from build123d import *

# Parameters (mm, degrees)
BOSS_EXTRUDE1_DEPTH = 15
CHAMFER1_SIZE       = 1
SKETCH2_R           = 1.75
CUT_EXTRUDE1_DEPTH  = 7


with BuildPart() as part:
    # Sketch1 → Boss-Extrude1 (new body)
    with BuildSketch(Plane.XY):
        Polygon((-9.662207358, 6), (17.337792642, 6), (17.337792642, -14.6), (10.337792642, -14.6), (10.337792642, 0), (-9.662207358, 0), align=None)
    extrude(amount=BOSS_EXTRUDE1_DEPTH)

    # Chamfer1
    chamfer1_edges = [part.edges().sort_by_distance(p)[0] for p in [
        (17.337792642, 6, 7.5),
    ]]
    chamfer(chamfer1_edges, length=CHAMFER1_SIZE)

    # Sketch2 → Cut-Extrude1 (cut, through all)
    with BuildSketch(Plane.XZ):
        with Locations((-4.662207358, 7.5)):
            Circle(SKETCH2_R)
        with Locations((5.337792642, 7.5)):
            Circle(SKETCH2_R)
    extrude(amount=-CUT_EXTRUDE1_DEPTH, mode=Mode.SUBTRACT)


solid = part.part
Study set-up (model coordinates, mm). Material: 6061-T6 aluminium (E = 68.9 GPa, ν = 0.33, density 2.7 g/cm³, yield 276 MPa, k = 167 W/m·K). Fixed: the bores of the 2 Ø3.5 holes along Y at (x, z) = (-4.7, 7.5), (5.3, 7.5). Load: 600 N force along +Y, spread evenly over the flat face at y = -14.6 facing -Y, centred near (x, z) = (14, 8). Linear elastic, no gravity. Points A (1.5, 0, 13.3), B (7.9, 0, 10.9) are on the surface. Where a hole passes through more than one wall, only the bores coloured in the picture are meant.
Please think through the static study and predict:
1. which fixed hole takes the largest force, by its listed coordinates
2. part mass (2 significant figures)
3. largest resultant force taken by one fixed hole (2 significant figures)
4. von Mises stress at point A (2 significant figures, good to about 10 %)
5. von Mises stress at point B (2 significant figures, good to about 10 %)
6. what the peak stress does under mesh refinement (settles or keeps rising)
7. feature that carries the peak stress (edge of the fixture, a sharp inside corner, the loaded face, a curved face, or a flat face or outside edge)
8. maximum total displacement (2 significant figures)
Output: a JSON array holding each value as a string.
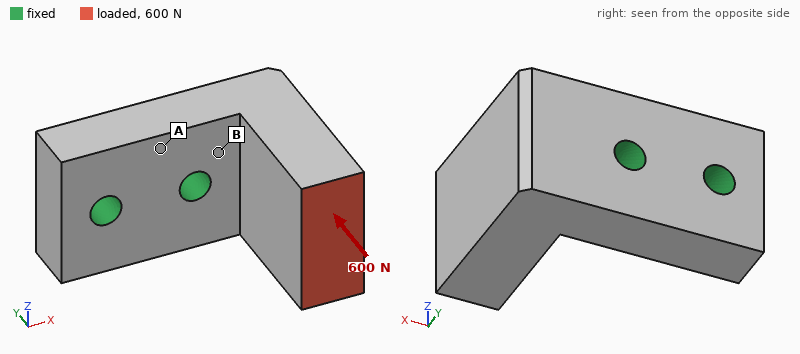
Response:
["(5.3, 7.5)", "10 g", "710 N", "11 MPa", "31 MPa", "keeps rising", "edge of the fixture", "27 µm"]
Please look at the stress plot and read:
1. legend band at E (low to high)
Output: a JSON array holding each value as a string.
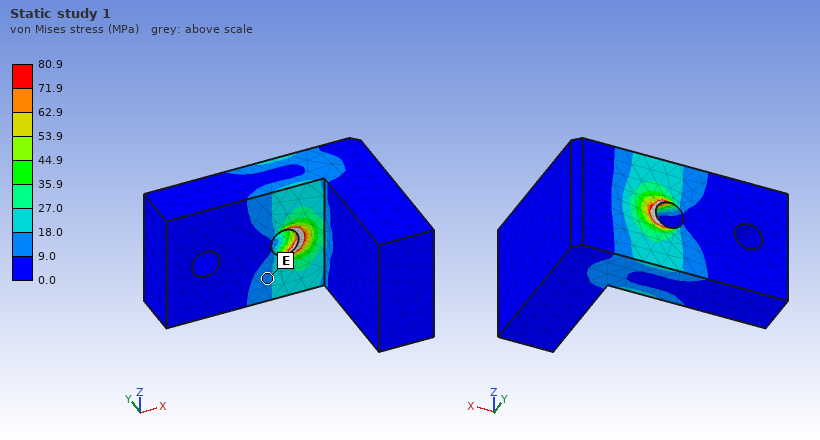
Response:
["9.0 to 18.0 MPa"]
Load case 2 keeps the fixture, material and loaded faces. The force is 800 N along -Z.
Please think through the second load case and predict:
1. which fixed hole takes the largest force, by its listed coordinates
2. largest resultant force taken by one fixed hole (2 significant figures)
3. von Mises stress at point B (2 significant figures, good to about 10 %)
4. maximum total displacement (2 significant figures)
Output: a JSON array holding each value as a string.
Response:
["(5.3, 7.5)", "1.2 kN", "130 MPa", "95 µm"]
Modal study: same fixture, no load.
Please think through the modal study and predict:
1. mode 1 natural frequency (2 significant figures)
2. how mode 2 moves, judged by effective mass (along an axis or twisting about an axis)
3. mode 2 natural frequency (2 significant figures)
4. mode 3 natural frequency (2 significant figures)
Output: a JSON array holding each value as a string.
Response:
["8700 Hz", "along Z", "11 kHz", "24 kHz"]
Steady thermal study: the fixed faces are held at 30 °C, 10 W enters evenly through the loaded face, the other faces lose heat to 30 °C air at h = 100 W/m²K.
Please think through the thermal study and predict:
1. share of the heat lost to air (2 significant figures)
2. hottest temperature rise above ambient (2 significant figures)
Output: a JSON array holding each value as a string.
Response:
["7.8 %", "13 K"]
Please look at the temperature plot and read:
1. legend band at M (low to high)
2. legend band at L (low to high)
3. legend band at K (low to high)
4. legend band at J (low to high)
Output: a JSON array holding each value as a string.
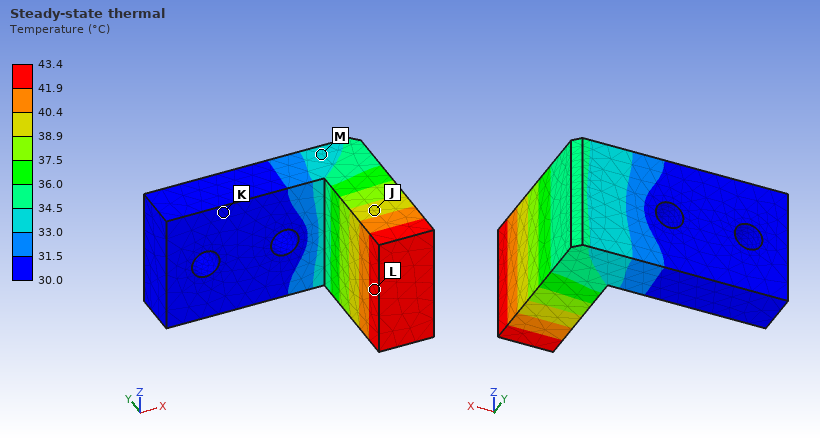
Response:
["33.0 to 34.5 °C", "41.9 to 43.4 °C", "30.0 to 31.5 °C", "38.9 to 40.4 °C"]
